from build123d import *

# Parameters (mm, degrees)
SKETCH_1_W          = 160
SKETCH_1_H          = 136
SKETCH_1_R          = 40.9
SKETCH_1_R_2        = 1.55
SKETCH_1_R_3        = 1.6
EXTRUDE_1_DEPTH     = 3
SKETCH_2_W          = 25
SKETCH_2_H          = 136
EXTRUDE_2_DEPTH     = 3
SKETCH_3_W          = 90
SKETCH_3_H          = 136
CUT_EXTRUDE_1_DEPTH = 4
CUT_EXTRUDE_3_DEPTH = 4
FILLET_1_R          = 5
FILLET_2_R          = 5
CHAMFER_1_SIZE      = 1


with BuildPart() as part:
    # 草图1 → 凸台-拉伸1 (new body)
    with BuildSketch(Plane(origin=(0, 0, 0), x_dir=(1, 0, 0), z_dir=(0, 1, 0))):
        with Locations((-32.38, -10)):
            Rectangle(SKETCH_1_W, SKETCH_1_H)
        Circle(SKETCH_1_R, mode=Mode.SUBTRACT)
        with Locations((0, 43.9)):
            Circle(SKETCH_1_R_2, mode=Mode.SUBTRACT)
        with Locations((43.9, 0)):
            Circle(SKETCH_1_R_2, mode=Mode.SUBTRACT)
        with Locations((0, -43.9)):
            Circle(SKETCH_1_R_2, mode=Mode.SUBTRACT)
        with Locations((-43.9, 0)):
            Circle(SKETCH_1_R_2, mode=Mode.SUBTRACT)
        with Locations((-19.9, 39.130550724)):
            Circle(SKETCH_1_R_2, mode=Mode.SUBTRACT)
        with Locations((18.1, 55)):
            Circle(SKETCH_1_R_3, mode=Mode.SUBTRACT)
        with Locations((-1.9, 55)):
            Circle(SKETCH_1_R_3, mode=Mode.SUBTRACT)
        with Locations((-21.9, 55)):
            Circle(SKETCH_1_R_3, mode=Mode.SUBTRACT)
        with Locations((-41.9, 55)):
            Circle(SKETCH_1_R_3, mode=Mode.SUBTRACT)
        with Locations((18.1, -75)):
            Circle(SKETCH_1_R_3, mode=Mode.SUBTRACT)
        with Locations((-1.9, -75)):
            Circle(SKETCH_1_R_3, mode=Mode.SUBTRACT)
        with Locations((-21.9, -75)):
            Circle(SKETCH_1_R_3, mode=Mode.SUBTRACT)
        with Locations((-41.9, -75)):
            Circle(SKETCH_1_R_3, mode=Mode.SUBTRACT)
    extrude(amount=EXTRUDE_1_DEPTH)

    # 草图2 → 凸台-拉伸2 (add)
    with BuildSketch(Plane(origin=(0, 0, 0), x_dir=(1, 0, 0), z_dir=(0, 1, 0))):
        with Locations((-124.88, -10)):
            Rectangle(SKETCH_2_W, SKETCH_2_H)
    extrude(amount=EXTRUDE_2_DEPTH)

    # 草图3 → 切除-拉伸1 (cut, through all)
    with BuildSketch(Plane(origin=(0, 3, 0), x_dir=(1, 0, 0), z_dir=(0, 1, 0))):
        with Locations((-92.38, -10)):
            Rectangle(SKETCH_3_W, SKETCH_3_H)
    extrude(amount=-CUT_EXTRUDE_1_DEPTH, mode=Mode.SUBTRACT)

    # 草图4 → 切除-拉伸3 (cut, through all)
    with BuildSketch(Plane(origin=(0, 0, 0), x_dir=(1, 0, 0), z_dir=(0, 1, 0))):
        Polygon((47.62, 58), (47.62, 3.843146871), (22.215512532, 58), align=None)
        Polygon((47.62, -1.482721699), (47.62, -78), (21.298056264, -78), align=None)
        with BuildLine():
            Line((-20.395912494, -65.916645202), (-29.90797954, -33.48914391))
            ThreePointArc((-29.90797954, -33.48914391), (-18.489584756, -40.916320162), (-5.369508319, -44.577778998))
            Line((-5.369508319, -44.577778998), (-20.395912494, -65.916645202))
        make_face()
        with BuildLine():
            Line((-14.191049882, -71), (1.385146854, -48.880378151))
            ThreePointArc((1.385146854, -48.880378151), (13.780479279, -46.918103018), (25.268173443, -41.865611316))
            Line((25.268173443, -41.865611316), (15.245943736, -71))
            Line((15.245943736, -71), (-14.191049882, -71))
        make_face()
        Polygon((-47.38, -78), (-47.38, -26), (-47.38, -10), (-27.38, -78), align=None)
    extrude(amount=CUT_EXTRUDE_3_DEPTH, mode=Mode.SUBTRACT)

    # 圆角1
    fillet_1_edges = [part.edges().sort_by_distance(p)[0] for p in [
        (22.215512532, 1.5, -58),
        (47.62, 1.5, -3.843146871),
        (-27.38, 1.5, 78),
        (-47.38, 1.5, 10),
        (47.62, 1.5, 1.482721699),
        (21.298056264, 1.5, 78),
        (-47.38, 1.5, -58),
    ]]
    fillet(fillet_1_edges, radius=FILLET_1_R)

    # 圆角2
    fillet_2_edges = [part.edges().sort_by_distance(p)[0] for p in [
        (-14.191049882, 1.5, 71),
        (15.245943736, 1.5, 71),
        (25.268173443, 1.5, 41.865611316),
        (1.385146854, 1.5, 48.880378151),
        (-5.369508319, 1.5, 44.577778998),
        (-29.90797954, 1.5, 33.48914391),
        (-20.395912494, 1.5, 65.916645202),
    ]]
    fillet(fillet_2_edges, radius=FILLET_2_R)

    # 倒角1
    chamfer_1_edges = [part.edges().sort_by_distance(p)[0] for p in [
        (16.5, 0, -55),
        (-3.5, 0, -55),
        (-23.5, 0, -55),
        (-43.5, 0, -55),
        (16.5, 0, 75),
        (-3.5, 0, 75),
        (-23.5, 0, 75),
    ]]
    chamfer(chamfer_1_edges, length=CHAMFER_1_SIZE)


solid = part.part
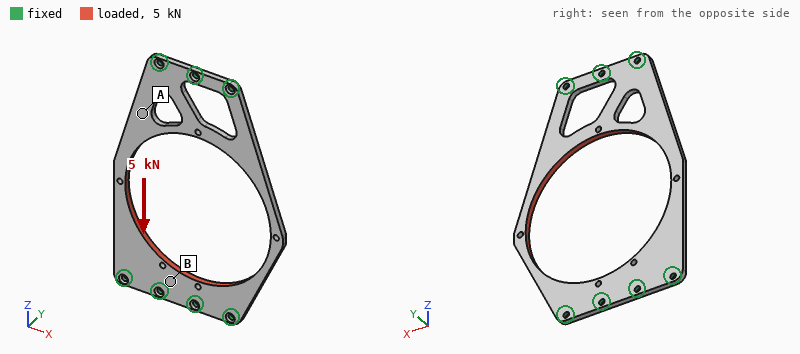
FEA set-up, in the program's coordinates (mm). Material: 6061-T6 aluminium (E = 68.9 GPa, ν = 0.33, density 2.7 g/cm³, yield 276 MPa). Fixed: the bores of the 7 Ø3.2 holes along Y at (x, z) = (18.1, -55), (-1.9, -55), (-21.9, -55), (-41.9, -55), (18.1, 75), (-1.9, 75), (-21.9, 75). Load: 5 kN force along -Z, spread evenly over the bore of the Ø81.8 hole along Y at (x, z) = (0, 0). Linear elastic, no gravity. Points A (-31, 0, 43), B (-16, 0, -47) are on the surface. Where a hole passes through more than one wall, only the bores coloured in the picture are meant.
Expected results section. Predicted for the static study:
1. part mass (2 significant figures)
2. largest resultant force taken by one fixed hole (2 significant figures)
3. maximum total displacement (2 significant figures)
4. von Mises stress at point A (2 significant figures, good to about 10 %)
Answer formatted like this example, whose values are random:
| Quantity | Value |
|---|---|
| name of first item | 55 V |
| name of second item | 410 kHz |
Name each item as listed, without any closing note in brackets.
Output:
| Quantity | Value |
|---|---|
| part mass | 35 g |
| largest resultant force taken by one fixed hole | 1.3 kN |
| maximum total displacement | 0.12 mm |
| von Mises stress at point A | 24 MPa |
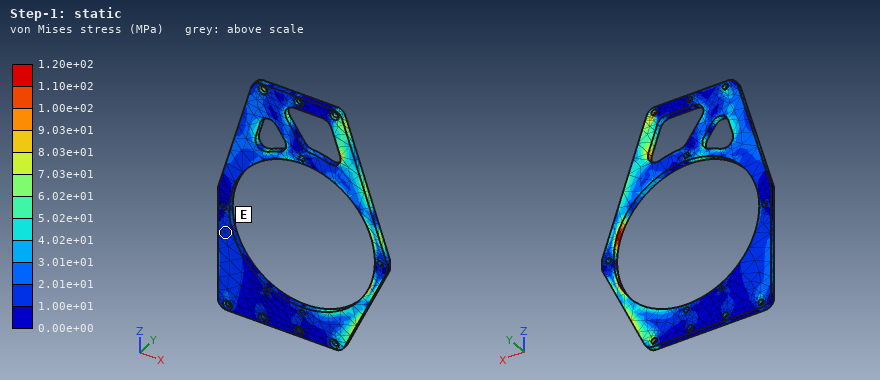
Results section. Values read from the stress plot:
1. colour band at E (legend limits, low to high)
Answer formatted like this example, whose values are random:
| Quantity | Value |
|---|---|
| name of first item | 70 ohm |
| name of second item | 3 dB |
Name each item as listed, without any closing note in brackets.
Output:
| Quantity | Value |
|---|---|
| colour band at E | 1.00e+01 to 2.01e+01 MPa |
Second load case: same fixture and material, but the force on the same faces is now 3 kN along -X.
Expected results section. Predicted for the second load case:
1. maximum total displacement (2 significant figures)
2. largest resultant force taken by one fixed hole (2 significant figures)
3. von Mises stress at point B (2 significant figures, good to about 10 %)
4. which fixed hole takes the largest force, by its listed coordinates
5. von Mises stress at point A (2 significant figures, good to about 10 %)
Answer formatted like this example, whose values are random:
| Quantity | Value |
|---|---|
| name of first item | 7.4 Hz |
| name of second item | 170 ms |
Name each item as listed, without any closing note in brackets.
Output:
| Quantity | Value |
|---|---|
| maximum total displacement | 0.13 mm |
| largest resultant force taken by one fixed hole | 910 N |
| von Mises stress at point B | 15 MPa |
| which fixed hole takes the largest force, by its listed coordinates | (-1.9, 75) |
| von Mises stress at point A | 28 MPa |
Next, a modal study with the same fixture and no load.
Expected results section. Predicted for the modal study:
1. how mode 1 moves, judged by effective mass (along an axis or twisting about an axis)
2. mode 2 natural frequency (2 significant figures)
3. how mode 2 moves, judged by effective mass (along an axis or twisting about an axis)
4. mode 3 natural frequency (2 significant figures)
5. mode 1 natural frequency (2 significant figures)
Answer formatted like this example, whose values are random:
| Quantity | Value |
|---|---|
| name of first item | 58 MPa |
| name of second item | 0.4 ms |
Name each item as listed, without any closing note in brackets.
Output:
| Quantity | Value |
|---|---|
| how mode 1 moves, judged by effective mass | along Y |
| mode 2 natural frequency | 1100 Hz |
| how mode 2 moves, judged by effective mass | along Y |
| mode 3 natural frequency | 2000 Hz |
| mode 1 natural frequency | 890 Hz |
